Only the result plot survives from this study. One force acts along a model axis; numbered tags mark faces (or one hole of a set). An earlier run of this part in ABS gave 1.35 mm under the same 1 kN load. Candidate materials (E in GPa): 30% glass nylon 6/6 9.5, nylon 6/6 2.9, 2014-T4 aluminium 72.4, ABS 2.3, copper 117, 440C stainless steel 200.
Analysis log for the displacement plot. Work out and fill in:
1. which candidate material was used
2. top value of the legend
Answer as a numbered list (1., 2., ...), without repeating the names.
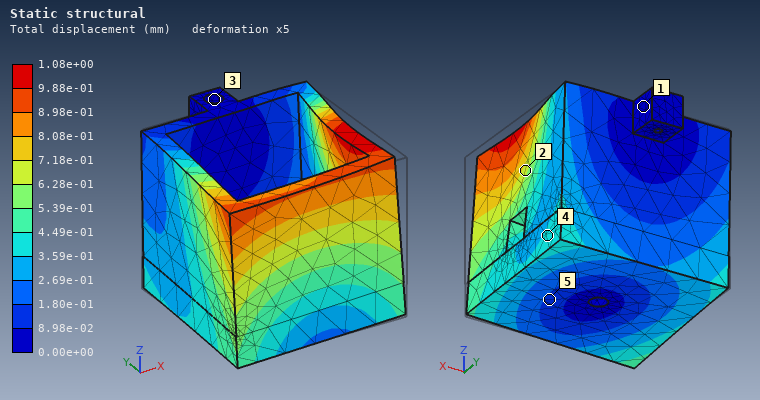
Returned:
1. nylon 6/6
2. 1.08e+00 mm
